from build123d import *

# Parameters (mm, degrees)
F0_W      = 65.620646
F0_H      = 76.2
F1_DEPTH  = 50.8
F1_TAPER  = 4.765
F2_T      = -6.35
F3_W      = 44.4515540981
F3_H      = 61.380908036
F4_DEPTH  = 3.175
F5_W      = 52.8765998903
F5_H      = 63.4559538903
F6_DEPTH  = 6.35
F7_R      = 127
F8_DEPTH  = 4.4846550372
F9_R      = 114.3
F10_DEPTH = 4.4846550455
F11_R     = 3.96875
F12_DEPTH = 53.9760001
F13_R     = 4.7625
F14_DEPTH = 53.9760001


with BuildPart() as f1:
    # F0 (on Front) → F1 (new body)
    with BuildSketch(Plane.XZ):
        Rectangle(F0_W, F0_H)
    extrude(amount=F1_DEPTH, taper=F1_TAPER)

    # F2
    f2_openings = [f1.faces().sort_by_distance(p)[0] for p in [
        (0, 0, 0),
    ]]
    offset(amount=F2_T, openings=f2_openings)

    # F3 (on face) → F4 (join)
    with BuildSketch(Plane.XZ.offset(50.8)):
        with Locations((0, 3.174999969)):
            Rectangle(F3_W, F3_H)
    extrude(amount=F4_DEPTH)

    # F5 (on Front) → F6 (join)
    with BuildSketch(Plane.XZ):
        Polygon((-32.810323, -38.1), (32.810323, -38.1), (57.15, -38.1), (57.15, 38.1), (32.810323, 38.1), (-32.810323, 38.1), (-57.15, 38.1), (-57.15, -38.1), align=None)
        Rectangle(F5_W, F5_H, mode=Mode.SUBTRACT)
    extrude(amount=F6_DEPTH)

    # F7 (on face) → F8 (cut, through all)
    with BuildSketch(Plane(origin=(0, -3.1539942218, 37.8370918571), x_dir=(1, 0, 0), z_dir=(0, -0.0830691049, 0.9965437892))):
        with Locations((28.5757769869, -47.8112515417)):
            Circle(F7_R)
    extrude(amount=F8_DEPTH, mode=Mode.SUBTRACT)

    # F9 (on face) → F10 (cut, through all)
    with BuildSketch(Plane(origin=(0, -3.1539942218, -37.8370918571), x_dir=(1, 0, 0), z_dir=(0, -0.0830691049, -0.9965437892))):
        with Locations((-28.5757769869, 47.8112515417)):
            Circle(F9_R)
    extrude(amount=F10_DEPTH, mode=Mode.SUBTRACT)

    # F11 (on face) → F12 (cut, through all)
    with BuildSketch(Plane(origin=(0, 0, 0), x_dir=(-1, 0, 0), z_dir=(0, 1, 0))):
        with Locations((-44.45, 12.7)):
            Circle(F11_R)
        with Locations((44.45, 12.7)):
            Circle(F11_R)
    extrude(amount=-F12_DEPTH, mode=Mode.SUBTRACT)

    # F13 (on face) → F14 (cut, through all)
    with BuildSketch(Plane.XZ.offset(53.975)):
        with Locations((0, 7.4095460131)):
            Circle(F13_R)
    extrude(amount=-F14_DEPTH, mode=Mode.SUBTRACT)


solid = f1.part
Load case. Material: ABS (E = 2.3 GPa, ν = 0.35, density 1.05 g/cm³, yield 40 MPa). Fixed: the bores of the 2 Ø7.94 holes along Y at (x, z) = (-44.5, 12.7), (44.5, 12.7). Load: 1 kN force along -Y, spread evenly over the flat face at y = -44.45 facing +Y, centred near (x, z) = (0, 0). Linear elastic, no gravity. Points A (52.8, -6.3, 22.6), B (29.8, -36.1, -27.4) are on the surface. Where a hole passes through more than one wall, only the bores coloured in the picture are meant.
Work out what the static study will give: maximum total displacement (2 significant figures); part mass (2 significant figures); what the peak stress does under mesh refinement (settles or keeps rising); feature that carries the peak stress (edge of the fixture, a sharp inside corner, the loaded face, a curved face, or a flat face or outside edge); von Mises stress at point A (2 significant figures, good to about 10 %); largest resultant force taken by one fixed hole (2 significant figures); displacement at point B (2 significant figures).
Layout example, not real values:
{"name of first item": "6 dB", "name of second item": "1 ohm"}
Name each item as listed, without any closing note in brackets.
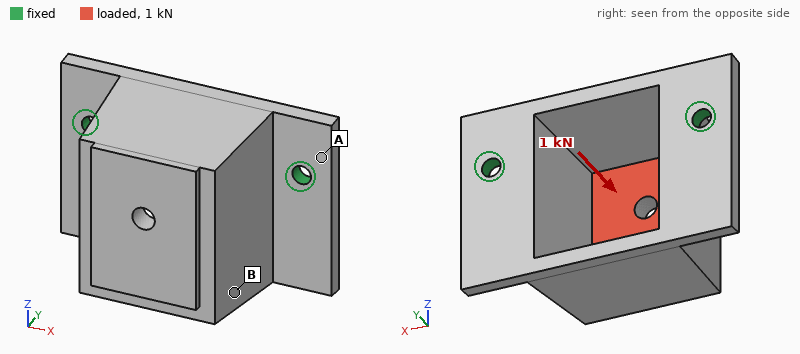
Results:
{"maximum total displacement": "1.5 mm", "part mass": "130 g", "what the peak stress does under mesh refinement": "keeps rising", "feature that carries the peak stress": "edge of the fixture", "von Mises stress at point A": "5.1 MPa", "largest resultant force taken by one fixed hole": "530 N", "displacement at point B": "1.2 mm"}
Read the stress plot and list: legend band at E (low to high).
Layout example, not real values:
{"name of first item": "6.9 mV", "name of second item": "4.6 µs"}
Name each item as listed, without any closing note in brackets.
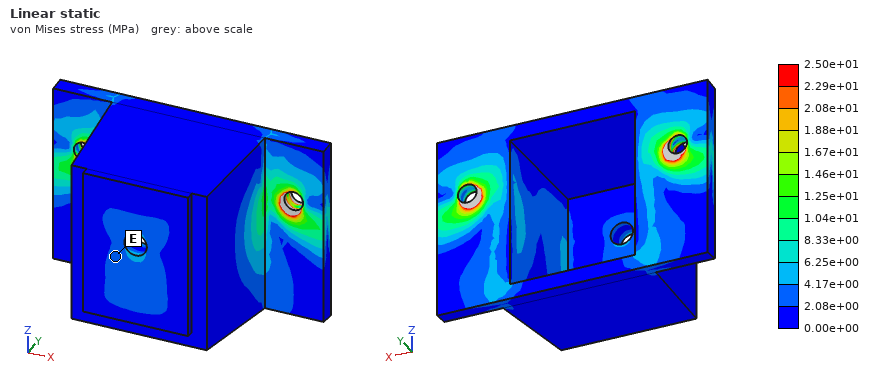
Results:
{"legend band at E": "2.08e+00 to 4.17e+00 MPa"}
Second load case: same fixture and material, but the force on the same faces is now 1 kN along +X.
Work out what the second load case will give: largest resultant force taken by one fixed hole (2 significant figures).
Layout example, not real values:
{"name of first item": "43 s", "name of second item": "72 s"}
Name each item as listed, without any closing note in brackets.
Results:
{"largest resultant force taken by one fixed hole": "750 N"}
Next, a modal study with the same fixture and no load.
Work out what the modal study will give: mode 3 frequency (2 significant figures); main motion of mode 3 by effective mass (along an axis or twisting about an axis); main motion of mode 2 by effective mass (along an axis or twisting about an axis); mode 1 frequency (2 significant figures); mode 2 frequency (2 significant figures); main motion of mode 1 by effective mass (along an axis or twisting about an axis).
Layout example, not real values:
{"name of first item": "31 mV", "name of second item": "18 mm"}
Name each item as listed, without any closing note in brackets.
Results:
{"mode 3 frequency": "1000 Hz", "main motion of mode 3 by effective mass": "twisting about Z", "main motion of mode 2 by effective mass": "along X", "mode 1 frequency": "280 Hz", "mode 2 frequency": "960 Hz", "main motion of mode 1 by effective mass": "along Z"}
